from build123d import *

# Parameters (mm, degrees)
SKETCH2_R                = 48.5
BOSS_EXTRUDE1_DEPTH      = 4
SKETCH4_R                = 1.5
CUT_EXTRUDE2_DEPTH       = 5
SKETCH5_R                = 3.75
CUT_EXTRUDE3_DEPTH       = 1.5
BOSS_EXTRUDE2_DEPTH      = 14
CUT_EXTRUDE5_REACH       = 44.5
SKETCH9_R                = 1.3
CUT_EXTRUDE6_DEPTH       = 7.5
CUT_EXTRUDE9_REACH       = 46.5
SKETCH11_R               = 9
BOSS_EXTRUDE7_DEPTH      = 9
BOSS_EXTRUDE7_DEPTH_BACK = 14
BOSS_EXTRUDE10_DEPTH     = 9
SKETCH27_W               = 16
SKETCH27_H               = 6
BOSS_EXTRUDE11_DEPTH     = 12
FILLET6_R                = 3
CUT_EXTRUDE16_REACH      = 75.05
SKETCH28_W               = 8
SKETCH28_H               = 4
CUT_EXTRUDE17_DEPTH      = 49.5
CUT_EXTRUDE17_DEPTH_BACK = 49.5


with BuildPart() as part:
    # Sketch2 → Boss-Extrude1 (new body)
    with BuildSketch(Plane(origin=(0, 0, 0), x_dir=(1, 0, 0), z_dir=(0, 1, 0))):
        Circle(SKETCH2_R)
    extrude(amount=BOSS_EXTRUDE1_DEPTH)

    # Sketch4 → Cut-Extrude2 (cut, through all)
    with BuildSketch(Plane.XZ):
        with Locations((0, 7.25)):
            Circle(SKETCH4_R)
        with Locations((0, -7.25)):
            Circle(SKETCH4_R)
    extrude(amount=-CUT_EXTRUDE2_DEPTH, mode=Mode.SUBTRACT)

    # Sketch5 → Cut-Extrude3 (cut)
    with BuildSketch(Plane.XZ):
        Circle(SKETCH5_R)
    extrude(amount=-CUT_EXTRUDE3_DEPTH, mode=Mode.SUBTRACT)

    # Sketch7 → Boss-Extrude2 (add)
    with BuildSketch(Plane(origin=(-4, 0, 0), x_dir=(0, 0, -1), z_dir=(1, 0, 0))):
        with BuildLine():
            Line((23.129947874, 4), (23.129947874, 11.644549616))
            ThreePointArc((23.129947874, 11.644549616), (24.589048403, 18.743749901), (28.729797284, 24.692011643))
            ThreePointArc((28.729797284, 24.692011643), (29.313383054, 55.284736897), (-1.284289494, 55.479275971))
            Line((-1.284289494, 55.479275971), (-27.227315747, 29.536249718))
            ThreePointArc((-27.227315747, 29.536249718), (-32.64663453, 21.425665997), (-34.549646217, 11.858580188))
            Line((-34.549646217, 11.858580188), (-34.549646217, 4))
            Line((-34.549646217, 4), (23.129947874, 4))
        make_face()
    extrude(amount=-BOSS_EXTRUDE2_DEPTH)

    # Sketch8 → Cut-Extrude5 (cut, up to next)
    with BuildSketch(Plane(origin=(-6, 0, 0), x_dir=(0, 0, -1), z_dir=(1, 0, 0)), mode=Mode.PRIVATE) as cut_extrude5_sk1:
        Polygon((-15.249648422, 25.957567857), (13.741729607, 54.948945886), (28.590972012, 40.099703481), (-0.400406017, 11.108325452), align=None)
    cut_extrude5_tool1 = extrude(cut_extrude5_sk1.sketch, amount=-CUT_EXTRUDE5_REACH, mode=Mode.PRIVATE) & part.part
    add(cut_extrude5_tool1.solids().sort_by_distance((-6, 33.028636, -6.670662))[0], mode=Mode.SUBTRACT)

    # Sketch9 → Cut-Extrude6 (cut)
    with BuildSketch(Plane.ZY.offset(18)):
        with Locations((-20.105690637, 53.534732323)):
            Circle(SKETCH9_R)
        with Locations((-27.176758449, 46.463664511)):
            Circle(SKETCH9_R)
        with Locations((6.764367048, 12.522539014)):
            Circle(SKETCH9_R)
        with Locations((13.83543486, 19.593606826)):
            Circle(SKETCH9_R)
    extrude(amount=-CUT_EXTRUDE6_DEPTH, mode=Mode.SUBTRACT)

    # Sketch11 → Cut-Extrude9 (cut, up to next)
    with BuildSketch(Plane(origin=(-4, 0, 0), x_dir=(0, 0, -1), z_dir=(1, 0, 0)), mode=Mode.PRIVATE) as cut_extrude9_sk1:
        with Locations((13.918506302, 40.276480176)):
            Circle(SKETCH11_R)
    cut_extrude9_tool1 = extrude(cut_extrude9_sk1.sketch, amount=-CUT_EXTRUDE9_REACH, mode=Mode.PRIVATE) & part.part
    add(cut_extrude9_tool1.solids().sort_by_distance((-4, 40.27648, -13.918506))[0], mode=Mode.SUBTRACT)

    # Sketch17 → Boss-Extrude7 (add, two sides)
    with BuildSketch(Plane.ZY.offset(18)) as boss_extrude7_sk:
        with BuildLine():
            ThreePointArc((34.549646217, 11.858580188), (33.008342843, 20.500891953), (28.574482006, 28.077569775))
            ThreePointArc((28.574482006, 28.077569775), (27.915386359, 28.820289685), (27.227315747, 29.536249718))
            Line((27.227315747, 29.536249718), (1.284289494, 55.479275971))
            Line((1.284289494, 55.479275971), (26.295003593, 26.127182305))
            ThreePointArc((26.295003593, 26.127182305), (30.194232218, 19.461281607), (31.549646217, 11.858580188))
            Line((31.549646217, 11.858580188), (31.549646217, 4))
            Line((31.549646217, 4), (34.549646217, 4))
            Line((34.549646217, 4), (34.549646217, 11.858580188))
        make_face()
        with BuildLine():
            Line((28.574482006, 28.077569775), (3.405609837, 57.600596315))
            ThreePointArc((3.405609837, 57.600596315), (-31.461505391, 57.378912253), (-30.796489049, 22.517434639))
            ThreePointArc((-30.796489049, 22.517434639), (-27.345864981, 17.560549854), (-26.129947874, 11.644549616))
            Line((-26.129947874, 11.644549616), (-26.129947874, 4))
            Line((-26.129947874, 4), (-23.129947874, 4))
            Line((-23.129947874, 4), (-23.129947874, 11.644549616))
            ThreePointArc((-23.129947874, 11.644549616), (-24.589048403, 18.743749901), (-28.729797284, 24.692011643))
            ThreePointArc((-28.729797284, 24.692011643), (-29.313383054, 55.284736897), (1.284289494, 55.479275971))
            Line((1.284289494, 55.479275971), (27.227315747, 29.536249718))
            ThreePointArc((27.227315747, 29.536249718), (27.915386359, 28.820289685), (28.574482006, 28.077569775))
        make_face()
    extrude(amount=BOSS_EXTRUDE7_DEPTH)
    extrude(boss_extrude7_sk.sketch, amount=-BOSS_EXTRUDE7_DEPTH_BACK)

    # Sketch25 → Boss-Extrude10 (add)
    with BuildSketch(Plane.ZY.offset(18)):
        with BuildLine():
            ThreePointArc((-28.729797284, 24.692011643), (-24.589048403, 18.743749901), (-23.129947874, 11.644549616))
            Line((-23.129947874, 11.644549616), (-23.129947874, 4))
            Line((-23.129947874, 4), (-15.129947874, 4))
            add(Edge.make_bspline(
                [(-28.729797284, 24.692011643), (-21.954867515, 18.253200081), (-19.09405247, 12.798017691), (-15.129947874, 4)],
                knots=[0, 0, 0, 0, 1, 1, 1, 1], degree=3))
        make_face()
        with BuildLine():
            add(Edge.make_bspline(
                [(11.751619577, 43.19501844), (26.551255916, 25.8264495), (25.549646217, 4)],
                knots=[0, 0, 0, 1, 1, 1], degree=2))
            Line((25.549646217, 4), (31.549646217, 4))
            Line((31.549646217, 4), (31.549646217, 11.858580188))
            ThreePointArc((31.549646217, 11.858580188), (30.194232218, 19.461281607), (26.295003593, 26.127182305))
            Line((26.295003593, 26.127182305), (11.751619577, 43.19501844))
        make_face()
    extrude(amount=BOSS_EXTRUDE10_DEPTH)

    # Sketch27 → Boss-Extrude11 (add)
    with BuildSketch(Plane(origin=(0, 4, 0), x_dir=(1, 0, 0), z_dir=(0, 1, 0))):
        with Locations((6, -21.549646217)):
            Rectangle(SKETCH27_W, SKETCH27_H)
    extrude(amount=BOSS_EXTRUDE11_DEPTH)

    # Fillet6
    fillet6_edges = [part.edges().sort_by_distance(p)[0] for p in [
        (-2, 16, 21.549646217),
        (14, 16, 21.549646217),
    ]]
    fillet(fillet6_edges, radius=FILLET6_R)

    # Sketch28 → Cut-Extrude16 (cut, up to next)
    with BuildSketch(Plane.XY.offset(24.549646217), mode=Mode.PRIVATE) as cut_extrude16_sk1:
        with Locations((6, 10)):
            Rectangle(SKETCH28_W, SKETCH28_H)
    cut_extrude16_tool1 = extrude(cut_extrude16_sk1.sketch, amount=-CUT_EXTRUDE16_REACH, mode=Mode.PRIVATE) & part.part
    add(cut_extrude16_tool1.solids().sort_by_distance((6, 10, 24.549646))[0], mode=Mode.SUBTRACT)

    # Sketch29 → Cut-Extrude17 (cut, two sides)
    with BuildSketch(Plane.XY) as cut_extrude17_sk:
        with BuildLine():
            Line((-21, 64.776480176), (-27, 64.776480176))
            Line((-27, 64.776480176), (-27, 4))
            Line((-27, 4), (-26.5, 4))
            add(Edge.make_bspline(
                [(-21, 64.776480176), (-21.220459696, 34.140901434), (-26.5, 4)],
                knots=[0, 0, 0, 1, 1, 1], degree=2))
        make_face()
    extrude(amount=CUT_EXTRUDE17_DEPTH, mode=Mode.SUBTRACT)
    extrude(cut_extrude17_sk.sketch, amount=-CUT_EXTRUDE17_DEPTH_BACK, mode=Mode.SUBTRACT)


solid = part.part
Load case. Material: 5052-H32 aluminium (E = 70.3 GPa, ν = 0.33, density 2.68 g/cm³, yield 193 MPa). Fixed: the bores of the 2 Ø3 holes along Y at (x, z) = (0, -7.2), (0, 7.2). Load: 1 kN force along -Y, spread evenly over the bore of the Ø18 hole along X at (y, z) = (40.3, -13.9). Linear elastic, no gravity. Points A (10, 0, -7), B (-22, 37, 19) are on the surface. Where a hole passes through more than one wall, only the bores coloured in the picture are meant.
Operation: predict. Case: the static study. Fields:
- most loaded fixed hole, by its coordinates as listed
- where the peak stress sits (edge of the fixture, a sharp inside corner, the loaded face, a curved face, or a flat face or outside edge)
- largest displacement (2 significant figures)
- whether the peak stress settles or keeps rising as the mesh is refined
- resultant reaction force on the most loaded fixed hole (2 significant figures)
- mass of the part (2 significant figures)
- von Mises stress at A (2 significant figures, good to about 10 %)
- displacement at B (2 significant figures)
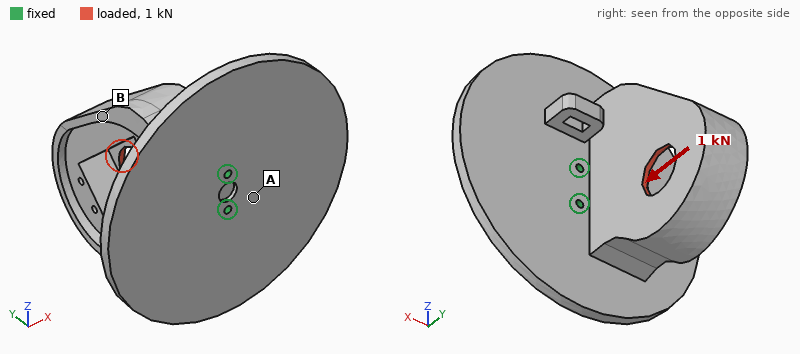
(0, -7.2)
edge of the fixture
90 µm
keeps rising
1.2 kN
180 g
7.1 MPa
41 µm
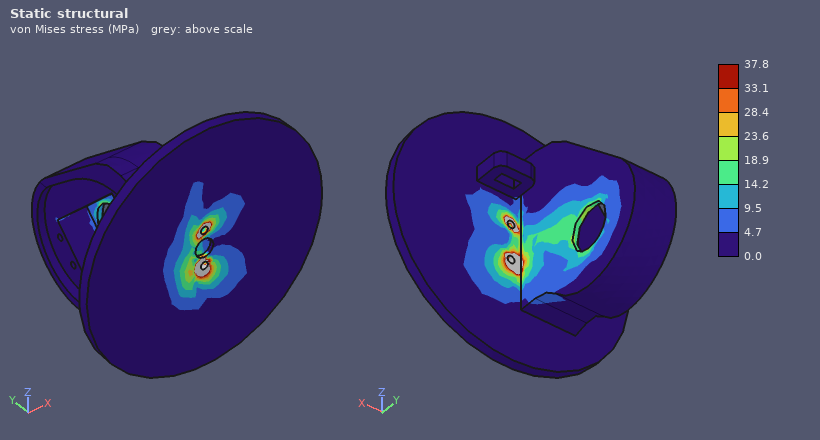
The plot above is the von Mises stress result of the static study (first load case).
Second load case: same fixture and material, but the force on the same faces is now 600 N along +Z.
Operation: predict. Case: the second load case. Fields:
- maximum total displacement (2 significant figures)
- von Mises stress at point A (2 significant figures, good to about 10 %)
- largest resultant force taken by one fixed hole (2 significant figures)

0.10 mm
12 MPa
1.3 kN
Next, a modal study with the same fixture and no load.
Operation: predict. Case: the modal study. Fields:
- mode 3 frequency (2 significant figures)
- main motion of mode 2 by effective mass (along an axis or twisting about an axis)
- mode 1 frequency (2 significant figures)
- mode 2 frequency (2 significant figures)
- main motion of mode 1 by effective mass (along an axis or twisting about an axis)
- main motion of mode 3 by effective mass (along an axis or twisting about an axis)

1700 Hz
along Z
650 Hz
1400 Hz
along X
along Y
